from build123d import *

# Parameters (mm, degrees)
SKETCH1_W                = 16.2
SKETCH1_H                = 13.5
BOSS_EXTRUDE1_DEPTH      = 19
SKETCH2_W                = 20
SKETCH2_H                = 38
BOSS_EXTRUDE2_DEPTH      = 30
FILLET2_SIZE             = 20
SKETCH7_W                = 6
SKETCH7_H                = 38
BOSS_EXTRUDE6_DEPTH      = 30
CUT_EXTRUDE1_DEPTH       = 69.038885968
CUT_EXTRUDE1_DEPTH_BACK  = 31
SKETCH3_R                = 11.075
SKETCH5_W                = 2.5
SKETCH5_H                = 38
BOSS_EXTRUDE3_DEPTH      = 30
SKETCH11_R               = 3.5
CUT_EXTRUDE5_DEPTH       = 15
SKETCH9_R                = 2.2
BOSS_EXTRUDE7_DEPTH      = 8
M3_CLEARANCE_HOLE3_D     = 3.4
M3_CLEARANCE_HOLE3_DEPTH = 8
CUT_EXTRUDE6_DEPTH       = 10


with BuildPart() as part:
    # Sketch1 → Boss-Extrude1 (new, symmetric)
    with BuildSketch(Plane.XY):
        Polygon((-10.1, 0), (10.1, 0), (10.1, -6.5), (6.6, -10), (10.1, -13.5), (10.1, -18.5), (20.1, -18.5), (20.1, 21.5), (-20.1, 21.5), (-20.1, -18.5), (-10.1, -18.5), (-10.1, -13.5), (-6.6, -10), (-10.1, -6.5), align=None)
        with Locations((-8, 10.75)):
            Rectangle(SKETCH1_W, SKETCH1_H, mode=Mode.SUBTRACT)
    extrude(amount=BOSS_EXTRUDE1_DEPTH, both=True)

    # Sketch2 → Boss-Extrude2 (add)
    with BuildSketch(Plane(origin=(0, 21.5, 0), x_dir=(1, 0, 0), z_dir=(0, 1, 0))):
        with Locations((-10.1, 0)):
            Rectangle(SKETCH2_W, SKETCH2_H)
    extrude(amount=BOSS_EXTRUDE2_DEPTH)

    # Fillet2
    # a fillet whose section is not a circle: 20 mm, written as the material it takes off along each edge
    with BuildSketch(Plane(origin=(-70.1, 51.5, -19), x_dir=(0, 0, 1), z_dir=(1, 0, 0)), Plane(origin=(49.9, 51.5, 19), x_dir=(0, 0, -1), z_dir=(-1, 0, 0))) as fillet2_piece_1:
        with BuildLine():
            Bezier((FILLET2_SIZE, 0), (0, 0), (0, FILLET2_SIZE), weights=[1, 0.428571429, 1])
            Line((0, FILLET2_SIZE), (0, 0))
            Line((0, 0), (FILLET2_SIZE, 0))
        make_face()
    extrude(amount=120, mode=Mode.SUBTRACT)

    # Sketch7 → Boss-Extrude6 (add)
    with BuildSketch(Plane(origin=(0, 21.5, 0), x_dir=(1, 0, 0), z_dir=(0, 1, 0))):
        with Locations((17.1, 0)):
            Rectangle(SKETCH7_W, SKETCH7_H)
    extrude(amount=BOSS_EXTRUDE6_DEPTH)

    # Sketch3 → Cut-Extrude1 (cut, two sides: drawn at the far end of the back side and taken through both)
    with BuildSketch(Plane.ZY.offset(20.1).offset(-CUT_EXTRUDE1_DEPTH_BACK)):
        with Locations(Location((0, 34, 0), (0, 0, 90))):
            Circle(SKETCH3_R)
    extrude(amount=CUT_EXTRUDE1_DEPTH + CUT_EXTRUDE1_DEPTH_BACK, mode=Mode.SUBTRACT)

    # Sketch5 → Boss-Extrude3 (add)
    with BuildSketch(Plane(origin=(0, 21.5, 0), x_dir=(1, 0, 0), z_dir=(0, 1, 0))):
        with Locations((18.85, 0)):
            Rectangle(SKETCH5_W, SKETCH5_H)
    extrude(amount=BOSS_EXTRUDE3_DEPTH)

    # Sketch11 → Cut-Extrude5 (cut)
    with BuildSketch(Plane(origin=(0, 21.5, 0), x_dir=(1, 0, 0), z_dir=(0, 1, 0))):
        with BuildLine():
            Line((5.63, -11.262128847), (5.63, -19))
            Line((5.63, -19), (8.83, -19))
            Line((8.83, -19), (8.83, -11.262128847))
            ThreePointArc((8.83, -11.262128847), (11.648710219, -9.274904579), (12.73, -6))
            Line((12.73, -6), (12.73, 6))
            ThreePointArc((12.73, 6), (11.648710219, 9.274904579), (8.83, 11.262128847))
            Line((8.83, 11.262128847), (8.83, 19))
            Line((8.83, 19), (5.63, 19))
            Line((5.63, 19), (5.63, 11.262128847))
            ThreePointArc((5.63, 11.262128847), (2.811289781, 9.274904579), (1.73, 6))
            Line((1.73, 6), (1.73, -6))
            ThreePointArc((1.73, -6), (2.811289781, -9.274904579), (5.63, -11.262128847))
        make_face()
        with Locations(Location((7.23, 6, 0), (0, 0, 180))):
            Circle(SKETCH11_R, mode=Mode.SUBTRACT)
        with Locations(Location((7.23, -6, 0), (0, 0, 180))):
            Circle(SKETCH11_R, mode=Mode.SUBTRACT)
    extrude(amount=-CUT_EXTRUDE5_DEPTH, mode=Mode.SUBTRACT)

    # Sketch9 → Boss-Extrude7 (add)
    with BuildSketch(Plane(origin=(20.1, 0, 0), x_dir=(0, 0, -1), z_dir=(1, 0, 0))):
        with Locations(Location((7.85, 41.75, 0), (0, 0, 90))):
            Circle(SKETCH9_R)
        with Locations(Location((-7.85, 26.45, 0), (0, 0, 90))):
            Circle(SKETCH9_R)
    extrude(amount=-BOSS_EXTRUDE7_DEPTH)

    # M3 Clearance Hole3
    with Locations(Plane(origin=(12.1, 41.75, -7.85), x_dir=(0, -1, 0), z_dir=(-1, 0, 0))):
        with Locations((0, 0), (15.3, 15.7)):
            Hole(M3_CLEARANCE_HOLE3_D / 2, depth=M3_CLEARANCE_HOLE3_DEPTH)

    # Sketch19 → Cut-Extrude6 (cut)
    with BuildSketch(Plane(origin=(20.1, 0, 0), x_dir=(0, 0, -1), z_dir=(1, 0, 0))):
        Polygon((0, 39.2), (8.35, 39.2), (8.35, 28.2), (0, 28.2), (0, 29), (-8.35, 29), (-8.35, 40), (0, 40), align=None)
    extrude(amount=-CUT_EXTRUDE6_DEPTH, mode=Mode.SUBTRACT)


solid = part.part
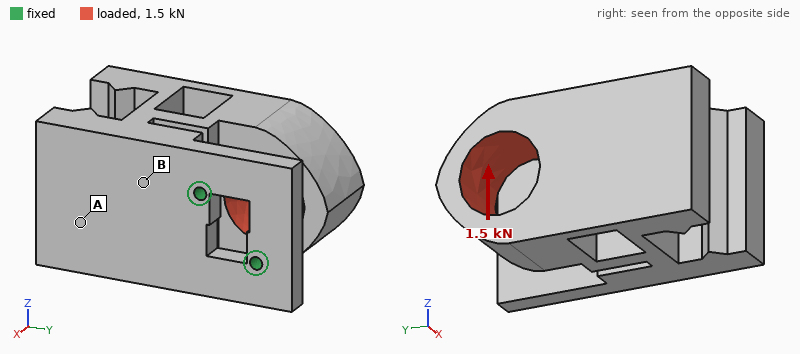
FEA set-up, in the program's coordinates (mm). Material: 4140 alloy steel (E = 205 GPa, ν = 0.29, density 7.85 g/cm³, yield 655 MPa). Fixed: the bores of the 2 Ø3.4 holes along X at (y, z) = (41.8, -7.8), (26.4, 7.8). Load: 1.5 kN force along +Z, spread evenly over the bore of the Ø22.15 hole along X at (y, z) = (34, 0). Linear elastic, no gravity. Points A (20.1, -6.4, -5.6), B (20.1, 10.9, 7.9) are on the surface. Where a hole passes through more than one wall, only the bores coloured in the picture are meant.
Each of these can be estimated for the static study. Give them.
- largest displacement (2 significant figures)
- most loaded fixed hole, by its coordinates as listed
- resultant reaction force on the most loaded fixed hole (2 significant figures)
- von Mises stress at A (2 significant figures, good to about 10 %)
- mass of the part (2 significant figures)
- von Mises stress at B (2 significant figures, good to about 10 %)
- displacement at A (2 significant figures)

0.17 mm
(26.4, 7.8)
1.6 kN
27 MPa
410 g
75 MPa
0.059 mm
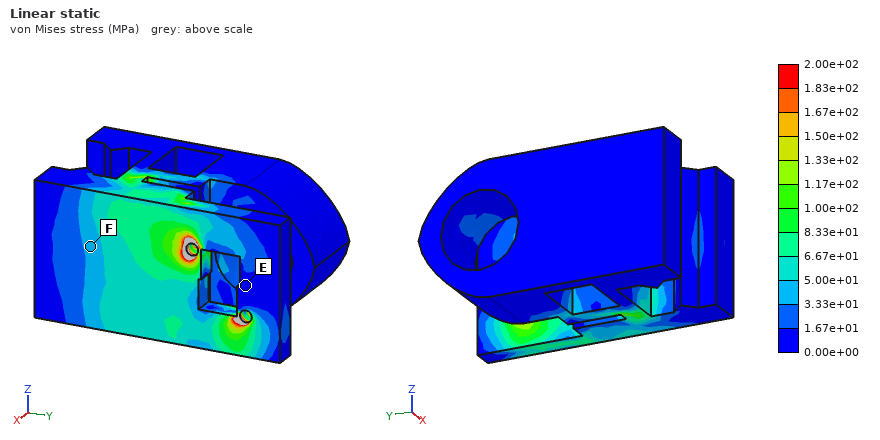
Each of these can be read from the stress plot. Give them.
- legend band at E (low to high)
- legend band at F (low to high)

0.00e+00 to 1.67e+01 MPa
3.33e+01 to 5.00e+01 MPa
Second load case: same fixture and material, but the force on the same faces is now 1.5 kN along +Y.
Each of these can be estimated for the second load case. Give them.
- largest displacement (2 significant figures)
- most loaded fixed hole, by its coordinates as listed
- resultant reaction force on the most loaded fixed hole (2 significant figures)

0.33 mm
(26.4, 7.8)
1.1 kN
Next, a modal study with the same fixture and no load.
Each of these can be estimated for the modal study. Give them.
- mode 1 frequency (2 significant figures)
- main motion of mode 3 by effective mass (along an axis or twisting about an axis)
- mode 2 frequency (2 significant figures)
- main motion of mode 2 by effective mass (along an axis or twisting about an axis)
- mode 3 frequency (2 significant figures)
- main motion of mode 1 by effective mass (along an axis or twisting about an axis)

710 Hz
along X
1200 Hz
along Z
1800 Hz
along Y
